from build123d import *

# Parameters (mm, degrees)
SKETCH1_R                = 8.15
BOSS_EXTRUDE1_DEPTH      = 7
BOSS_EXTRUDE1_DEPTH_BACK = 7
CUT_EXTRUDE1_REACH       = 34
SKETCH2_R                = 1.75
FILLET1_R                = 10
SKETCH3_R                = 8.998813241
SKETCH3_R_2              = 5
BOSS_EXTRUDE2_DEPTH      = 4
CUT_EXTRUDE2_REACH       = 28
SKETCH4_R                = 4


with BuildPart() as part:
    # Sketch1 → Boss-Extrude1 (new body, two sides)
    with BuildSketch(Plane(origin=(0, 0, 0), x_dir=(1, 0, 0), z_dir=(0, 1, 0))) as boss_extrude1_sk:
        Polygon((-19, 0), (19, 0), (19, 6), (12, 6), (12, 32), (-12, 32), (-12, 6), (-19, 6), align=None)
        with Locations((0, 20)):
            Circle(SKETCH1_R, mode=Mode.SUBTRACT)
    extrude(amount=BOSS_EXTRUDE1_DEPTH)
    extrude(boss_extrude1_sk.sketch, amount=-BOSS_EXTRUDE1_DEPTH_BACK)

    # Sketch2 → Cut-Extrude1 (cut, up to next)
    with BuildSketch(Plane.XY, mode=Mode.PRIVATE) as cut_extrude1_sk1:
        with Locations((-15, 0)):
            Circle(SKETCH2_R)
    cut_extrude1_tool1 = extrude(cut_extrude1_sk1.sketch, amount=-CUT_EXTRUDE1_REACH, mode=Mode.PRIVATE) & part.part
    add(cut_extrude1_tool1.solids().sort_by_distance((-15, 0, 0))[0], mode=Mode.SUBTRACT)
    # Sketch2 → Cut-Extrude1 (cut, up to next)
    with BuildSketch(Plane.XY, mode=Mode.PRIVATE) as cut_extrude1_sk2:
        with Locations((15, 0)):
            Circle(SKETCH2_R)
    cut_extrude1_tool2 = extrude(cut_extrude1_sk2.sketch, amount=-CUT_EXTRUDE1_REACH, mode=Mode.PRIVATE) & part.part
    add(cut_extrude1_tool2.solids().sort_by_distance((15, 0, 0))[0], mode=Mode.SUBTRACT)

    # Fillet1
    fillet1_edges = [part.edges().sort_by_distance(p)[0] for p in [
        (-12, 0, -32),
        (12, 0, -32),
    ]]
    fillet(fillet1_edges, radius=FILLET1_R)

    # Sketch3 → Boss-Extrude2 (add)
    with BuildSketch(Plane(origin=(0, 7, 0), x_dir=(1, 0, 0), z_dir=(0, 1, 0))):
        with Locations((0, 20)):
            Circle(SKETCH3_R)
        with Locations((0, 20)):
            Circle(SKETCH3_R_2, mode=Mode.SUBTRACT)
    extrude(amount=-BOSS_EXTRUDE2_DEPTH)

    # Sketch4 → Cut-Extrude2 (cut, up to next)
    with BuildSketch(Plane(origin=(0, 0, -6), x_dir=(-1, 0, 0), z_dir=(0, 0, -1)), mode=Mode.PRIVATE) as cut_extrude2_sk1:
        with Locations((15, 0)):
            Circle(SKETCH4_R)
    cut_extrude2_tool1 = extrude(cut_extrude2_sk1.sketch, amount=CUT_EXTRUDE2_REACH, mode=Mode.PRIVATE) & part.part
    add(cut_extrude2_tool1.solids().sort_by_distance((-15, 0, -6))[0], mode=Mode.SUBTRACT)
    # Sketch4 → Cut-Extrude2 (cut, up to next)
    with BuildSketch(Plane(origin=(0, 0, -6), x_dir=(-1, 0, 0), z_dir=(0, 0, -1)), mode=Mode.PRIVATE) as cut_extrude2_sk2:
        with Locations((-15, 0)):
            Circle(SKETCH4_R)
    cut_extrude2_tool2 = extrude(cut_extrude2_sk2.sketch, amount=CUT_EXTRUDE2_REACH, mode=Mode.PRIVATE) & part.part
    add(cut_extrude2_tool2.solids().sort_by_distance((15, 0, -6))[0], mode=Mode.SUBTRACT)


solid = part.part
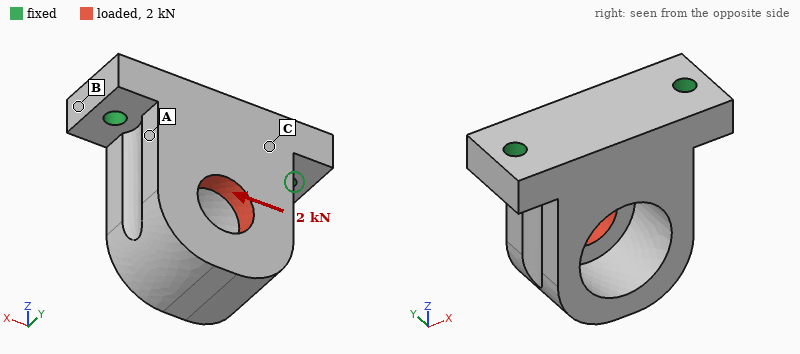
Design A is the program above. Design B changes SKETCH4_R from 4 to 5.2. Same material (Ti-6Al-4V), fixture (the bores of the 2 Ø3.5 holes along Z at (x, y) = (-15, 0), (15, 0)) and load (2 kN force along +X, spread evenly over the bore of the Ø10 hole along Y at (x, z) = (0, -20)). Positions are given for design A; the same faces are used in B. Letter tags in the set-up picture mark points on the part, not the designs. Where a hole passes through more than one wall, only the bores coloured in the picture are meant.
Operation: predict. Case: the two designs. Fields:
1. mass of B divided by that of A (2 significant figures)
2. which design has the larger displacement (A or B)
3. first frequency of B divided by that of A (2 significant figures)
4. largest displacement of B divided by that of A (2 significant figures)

0.96
B
0.99
1.2
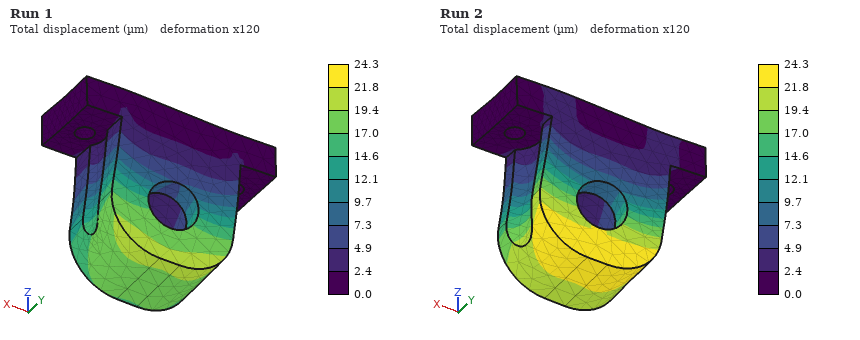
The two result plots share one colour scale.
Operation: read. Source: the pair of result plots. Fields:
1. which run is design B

Run 2
